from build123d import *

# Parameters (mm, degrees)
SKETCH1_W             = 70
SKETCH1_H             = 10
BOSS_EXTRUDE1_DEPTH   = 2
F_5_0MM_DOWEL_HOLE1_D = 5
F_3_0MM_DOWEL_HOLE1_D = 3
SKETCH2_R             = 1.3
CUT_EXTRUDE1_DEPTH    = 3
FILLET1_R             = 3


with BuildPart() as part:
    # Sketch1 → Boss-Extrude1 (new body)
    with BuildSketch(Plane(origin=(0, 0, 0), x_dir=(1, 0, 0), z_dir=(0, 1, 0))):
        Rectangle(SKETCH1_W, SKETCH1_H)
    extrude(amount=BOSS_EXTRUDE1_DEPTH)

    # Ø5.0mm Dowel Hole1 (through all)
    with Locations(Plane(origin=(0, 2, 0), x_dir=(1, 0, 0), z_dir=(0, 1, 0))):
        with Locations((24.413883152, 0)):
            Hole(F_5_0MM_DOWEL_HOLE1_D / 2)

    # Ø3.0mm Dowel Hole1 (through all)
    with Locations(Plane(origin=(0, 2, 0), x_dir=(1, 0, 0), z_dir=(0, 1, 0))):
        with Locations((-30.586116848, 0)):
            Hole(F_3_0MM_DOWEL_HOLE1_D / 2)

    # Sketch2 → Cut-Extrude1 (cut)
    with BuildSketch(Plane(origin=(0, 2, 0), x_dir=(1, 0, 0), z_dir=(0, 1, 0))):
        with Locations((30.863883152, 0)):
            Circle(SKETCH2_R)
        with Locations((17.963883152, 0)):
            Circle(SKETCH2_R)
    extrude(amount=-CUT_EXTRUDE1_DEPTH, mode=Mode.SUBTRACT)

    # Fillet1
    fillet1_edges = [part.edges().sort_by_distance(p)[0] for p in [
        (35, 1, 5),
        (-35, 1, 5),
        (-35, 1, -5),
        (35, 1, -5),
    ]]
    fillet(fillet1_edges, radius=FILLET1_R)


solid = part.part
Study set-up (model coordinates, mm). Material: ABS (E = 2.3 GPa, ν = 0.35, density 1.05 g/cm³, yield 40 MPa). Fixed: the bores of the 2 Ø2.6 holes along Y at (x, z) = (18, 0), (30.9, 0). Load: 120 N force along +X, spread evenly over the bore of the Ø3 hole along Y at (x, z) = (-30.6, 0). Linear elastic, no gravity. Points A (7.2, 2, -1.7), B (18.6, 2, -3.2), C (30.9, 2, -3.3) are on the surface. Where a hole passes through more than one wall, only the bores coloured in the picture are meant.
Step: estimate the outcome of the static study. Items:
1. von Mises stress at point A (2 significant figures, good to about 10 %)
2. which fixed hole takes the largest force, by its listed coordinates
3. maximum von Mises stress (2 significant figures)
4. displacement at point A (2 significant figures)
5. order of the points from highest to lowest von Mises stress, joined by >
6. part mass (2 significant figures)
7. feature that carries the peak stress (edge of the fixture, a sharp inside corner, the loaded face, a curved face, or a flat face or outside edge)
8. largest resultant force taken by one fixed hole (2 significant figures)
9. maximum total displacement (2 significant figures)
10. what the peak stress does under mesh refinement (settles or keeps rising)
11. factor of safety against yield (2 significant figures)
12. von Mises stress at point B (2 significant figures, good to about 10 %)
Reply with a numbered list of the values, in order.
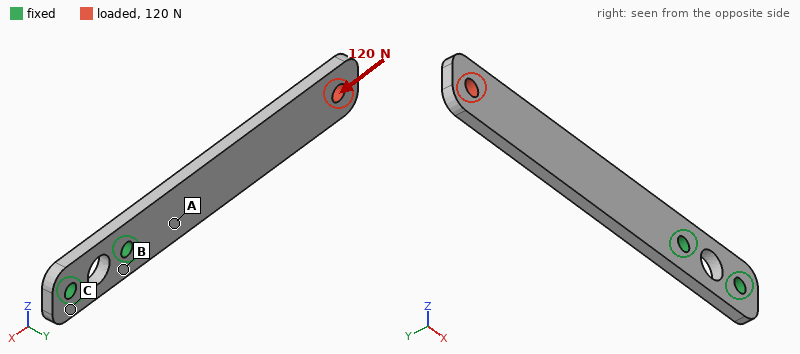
1. 6.1 MPa
2. (18, 0)
3. 17 MPa
4. 0.031 mm
5. A > B > C
6. 1.4 g
7. the loaded face
8. 110 N
9. 0.15 mm
10. settles
11. 2.4
12. 2.9 MPa
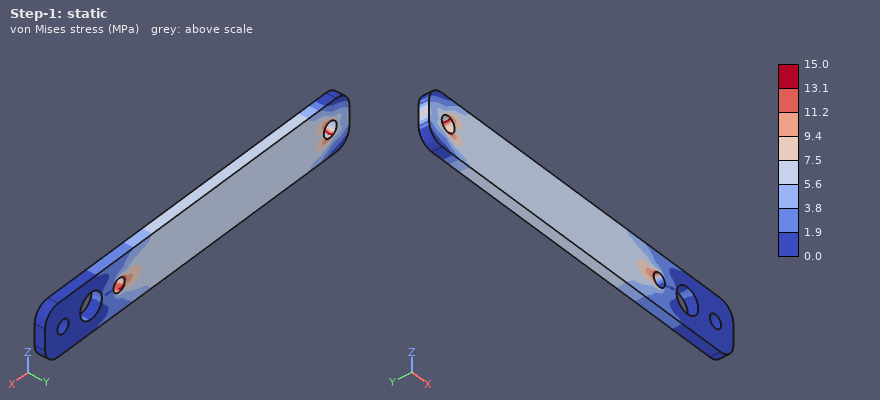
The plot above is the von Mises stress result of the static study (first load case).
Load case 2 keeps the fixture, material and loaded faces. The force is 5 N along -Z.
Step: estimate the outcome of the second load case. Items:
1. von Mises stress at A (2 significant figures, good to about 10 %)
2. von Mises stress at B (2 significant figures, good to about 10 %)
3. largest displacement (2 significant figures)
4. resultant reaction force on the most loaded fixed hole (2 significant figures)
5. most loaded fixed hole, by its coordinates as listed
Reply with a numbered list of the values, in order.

1. 2.0 MPa
2. 3.2 MPa
3. 0.74 mm
4. 13 N
5. (18, 0)
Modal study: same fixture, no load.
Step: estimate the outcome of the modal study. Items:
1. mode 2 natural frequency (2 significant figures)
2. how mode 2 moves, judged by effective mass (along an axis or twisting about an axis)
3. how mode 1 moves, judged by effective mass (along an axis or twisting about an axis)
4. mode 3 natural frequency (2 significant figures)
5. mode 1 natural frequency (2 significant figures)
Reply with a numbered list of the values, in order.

1. 740 Hz
2. along Z
3. along Y
4. 1100 Hz
5. 180 Hz
